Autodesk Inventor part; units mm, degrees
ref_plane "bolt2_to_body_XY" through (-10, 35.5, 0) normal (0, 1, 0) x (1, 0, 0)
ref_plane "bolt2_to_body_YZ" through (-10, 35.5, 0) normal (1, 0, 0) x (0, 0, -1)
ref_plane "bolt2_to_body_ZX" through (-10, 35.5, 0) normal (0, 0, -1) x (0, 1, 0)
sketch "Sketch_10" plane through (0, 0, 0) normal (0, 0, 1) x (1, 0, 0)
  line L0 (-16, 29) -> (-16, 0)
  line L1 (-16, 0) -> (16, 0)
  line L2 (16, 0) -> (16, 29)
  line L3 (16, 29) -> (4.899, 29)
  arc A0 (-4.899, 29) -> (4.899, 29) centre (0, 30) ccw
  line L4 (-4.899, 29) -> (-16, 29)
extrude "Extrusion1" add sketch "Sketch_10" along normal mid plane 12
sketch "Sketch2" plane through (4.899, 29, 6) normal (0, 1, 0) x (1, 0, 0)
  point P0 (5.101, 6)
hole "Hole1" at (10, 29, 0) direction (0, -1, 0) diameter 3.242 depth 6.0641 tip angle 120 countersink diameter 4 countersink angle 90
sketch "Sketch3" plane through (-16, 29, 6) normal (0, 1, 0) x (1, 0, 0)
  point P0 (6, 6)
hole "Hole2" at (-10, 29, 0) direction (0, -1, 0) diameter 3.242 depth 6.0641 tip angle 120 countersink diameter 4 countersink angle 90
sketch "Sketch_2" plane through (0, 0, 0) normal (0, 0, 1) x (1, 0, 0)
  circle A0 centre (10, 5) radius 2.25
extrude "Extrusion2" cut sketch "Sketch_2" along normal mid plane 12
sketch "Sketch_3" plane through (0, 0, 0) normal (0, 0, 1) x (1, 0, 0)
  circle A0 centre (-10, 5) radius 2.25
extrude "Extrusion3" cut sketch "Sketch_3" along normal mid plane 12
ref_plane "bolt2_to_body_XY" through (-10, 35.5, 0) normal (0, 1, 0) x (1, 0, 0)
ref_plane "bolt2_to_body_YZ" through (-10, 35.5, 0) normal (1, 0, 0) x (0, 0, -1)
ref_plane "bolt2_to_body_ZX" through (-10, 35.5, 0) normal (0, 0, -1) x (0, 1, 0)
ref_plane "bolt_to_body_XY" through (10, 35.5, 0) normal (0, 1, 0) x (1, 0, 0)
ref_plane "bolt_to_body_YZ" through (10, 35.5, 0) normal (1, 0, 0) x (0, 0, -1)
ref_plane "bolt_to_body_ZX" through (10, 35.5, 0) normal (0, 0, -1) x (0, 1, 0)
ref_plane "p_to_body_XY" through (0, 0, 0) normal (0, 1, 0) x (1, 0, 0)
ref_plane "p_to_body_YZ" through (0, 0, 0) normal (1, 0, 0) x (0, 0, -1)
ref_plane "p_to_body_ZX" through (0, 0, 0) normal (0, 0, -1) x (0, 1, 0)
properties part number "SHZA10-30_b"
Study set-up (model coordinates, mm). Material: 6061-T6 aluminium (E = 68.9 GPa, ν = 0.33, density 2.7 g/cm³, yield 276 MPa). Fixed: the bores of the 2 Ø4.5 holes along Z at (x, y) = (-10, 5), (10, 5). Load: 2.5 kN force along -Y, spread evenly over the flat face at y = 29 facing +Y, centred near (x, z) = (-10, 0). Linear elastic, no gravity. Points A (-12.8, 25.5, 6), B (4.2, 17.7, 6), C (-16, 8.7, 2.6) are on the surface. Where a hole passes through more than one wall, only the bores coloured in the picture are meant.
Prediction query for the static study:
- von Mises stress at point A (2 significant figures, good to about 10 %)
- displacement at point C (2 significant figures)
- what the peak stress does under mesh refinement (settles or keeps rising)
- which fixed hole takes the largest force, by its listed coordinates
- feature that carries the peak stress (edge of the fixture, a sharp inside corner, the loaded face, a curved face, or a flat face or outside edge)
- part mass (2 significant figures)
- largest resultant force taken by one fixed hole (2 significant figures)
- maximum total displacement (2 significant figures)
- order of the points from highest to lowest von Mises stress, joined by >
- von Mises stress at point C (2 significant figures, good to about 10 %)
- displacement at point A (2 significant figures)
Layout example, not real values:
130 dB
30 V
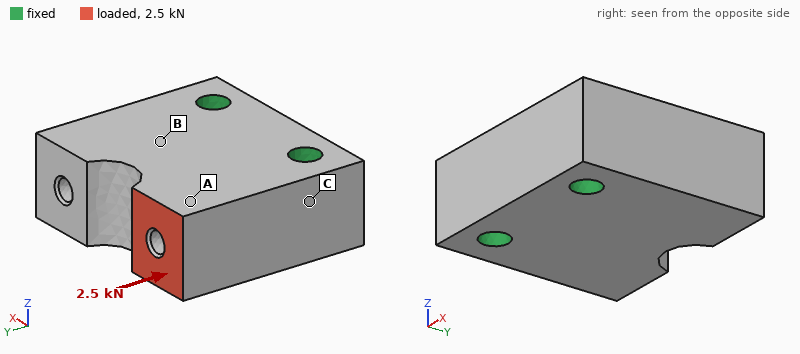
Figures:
21 MPa
1.9 µm
keeps rising
(-10, 5)
edge of the fixture
28 g
2.4 kN
9.5 µm
A > C > B
13 MPa
7.0 µm
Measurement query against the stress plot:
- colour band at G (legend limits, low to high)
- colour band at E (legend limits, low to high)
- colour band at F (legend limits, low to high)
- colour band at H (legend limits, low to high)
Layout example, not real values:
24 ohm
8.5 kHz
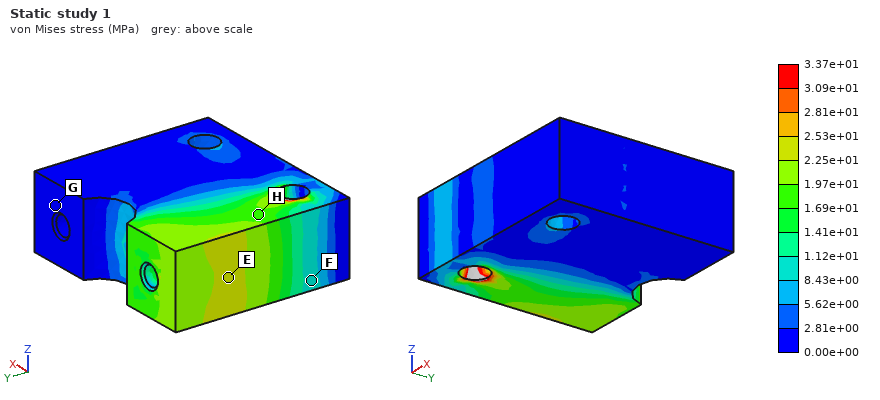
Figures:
0.00e+00 to 2.81e+00 MPa
2.25e+01 to 2.53e+01 MPa
8.43e+00 to 1.12e+01 MPa
1.69e+01 to 1.97e+01 MPa
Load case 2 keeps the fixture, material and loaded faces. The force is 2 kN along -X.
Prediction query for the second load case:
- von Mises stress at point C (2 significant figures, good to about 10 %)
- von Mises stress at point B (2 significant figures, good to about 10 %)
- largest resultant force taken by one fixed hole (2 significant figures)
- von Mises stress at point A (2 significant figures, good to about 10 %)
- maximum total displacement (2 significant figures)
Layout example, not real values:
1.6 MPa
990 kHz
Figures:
19 MPa
19 MPa
2.4 kN
17 MPa
22 µm
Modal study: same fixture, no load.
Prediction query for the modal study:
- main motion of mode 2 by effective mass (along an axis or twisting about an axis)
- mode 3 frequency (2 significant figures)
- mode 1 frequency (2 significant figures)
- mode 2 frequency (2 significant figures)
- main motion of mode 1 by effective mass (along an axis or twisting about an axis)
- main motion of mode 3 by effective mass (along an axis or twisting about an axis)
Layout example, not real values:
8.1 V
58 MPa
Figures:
twisting about Y
25 kHz
15 kHz
24 kHz
along Z
along X
